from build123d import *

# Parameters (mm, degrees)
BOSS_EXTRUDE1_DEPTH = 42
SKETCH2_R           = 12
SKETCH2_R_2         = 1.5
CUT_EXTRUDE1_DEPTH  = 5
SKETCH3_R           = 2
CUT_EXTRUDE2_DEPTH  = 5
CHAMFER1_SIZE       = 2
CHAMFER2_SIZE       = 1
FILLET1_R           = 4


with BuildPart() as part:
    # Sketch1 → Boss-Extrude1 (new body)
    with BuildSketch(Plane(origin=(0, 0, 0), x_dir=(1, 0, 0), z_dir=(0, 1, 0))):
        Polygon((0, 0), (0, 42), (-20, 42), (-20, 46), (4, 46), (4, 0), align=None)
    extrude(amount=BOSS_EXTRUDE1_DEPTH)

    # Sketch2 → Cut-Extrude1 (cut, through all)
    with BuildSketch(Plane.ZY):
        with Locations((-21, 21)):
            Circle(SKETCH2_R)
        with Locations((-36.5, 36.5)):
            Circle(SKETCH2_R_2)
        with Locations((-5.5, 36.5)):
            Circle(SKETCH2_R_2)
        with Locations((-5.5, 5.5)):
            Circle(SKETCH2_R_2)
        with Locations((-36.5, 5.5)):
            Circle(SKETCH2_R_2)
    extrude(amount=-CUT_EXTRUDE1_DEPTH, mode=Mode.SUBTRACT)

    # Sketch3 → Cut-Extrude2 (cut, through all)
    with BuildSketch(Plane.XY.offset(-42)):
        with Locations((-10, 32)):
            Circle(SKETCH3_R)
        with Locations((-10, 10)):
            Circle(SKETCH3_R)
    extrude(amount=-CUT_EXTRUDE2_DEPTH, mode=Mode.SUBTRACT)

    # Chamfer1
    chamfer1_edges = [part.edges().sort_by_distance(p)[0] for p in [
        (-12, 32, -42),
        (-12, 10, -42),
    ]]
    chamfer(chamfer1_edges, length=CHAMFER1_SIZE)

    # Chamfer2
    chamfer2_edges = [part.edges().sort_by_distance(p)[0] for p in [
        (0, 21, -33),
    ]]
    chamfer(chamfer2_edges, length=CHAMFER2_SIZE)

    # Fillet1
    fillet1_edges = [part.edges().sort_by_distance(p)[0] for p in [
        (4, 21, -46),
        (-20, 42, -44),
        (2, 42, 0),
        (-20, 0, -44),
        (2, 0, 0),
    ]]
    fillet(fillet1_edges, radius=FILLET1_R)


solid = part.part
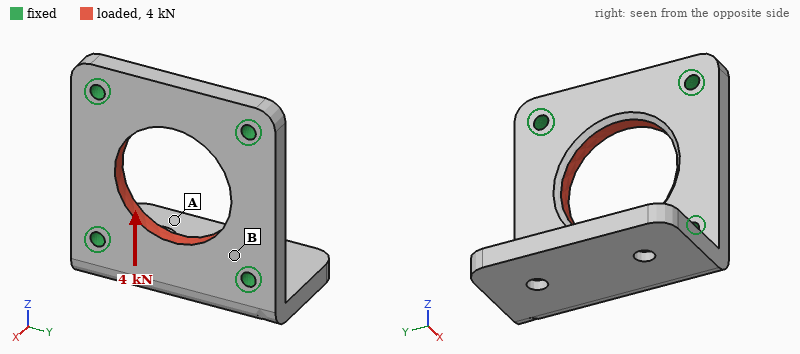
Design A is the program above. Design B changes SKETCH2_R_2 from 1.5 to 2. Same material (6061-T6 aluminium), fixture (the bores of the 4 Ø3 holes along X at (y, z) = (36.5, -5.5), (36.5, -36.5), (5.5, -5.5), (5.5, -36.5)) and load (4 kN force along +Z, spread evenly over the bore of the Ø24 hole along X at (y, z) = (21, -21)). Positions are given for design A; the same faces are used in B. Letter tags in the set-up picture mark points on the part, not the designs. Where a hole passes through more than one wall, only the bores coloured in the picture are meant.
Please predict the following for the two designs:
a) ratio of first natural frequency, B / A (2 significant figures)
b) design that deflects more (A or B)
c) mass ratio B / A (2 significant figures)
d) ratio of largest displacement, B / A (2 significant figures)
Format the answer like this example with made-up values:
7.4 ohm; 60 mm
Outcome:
1.0; A; 0.99; 0.91
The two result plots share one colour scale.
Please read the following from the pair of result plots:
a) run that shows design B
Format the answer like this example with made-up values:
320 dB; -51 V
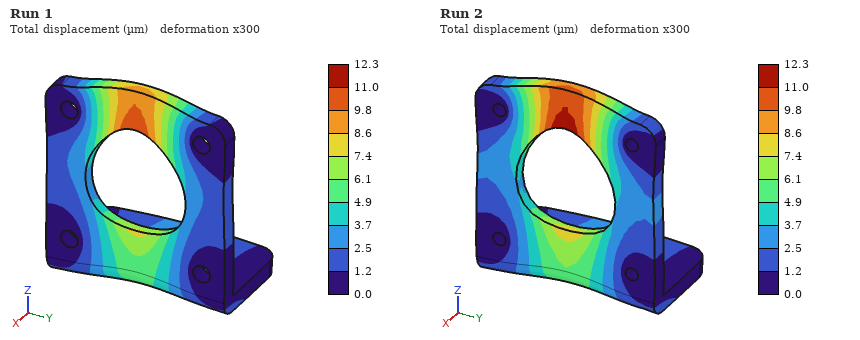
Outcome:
Run 1
